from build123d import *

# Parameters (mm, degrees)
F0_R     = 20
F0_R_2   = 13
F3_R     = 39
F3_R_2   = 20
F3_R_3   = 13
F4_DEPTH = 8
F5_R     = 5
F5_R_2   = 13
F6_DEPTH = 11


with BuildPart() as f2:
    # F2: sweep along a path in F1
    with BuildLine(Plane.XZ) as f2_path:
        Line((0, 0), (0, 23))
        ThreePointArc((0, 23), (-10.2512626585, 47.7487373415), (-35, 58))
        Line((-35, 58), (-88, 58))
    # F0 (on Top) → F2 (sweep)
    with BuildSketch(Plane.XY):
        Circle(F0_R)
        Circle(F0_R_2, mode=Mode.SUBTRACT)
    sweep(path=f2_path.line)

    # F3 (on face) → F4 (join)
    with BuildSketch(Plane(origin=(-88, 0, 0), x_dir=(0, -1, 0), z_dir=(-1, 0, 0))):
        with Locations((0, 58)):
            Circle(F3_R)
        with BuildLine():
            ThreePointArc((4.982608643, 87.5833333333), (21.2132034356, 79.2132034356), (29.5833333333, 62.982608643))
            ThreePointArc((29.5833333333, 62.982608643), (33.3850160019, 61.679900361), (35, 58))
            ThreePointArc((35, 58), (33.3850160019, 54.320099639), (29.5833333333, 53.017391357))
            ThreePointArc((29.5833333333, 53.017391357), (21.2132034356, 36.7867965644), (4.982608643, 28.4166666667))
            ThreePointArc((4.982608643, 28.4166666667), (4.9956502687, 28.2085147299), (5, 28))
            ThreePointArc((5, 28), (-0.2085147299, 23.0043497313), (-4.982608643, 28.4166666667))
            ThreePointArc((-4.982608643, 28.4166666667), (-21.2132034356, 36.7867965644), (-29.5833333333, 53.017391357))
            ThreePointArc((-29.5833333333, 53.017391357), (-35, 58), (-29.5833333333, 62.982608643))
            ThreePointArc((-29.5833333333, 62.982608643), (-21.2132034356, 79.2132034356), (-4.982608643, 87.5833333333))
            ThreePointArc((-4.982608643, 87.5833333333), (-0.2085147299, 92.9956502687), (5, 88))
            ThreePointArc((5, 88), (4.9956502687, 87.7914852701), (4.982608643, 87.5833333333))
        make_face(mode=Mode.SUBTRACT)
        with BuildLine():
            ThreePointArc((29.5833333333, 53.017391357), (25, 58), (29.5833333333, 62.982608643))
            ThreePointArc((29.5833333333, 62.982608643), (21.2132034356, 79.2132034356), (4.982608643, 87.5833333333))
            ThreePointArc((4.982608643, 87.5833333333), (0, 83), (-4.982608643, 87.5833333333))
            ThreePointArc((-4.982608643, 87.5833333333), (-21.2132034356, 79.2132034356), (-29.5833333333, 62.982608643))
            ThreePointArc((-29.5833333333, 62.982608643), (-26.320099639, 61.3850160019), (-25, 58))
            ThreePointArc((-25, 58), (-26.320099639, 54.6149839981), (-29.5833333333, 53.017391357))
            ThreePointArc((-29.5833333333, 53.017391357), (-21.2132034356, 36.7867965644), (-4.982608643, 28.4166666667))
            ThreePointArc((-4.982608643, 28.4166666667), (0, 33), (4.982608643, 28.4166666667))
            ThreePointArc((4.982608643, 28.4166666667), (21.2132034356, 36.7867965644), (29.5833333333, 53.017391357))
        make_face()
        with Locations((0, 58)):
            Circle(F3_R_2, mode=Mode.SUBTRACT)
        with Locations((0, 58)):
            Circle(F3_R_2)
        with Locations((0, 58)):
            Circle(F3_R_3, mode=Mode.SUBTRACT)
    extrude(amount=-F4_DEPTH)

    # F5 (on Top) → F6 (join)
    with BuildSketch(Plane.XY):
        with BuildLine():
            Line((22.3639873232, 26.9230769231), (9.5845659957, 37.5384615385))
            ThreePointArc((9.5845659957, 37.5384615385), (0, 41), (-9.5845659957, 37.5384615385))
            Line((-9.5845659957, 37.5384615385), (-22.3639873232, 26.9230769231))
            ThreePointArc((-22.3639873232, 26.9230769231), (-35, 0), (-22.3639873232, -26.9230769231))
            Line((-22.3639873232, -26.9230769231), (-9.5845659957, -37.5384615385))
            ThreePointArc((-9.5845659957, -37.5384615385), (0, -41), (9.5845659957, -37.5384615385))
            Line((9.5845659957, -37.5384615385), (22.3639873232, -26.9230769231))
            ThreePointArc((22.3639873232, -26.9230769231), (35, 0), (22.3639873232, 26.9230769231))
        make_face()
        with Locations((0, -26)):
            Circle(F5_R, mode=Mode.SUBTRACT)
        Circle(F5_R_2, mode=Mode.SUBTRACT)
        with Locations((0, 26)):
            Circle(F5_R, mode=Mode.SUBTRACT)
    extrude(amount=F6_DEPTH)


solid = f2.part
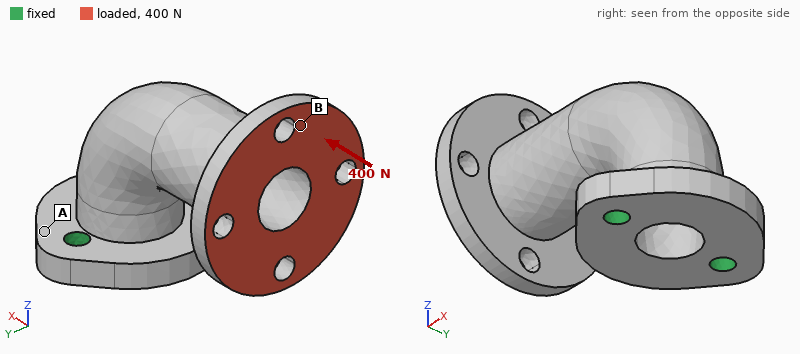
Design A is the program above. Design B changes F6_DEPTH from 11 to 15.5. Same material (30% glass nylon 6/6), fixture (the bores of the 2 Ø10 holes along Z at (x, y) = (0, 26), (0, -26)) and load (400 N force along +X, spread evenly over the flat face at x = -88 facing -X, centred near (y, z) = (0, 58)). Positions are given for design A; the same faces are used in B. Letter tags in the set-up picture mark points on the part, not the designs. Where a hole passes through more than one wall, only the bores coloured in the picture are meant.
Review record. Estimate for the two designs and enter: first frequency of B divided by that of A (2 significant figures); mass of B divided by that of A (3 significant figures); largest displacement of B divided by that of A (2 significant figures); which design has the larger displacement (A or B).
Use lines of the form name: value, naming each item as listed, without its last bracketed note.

first frequency of B divided by that of A: 1.2
mass of B divided by that of A: 1.08
largest displacement of B divided by that of A: 0.60
which design has the larger displacement: A
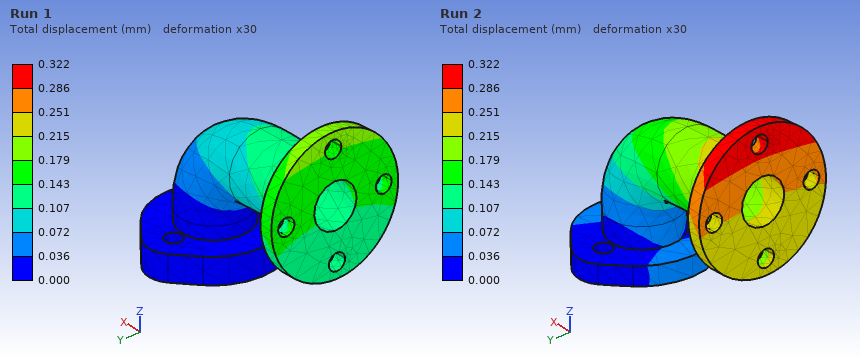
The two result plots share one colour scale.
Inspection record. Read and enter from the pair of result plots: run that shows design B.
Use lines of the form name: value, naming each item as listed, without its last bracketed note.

run that shows design B: Run 1
